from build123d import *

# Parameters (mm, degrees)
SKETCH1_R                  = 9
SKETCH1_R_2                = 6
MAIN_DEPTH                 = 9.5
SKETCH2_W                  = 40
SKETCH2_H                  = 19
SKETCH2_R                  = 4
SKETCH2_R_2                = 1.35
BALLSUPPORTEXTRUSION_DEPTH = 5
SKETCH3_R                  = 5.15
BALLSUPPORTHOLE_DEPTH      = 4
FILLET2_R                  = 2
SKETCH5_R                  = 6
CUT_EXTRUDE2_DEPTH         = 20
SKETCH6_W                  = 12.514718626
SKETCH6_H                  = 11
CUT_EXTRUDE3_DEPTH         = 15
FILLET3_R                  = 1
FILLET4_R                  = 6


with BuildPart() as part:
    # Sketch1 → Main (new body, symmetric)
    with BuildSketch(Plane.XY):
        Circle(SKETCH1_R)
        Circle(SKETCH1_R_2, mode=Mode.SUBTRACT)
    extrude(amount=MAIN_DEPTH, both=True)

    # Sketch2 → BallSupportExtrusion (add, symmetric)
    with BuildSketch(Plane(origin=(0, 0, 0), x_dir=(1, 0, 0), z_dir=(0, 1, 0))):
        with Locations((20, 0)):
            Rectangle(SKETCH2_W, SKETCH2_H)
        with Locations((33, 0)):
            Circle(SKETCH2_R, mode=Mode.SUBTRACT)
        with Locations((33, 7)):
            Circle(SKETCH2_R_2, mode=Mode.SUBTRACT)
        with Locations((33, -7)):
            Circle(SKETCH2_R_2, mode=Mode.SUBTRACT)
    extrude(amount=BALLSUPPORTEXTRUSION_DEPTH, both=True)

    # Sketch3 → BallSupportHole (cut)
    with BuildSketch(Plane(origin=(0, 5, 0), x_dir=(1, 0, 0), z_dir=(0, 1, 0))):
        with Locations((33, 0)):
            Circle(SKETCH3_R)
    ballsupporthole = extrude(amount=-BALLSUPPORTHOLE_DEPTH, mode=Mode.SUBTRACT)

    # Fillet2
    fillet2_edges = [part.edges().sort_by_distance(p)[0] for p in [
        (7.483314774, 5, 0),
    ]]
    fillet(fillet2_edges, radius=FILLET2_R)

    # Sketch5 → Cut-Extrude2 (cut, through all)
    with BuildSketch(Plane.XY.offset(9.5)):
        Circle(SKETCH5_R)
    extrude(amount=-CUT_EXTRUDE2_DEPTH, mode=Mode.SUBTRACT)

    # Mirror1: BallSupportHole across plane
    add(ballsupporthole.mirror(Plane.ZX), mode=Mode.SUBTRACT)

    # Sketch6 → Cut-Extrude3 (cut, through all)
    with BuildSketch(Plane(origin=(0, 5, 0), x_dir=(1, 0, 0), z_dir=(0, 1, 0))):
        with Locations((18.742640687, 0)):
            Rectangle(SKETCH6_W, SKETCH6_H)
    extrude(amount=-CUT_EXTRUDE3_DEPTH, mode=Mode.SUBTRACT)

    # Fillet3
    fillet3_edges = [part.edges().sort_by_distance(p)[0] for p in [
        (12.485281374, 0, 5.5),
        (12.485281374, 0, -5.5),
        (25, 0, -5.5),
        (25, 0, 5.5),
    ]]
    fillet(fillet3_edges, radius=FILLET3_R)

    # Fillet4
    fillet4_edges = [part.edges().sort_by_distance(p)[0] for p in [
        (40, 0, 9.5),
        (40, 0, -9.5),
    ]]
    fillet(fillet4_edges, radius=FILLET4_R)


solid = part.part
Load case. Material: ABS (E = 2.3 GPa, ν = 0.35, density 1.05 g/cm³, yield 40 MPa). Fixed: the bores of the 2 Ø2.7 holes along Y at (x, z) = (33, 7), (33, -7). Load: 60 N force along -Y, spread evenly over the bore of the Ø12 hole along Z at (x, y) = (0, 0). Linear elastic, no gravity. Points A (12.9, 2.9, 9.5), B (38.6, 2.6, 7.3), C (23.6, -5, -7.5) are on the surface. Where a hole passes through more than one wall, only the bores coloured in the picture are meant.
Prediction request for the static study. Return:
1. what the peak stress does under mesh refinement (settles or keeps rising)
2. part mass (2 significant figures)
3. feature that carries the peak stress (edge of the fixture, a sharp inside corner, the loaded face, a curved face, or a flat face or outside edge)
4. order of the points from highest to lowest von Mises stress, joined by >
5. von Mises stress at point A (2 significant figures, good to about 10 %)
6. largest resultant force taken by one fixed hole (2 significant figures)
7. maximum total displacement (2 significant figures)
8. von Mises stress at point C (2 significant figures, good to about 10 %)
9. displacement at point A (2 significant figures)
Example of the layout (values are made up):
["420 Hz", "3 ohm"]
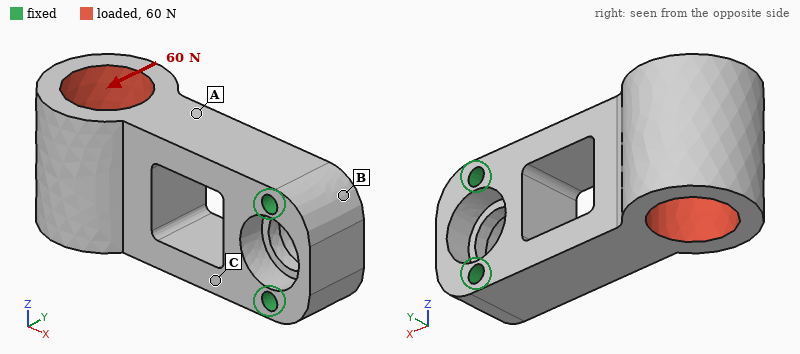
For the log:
["keeps rising", "6.6 g", "edge of the fixture", "C > A > B", "3.4 MPa", "30 N", "0.63 mm", "10.0 MPa", "0.18 mm"]
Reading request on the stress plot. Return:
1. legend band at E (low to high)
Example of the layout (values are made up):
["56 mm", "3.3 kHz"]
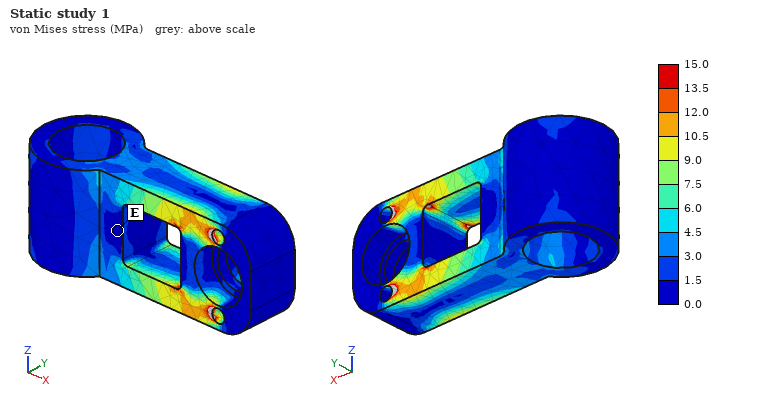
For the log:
["0.0 to 1.5 MPa"]
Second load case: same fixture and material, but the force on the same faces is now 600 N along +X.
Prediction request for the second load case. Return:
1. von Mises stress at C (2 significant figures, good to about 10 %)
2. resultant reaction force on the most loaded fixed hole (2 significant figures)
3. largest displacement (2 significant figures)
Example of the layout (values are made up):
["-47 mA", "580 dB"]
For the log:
["7.0 MPa", "300 N", "0.19 mm"]
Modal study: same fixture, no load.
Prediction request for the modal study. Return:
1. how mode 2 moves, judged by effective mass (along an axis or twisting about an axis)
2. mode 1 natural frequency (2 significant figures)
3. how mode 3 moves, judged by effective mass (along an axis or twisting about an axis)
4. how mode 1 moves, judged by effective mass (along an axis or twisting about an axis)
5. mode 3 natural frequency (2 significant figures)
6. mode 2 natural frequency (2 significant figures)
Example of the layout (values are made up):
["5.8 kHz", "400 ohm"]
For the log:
["along Z", "990 Hz", "twisting about X", "along Y", "2800 Hz", "1500 Hz"]
